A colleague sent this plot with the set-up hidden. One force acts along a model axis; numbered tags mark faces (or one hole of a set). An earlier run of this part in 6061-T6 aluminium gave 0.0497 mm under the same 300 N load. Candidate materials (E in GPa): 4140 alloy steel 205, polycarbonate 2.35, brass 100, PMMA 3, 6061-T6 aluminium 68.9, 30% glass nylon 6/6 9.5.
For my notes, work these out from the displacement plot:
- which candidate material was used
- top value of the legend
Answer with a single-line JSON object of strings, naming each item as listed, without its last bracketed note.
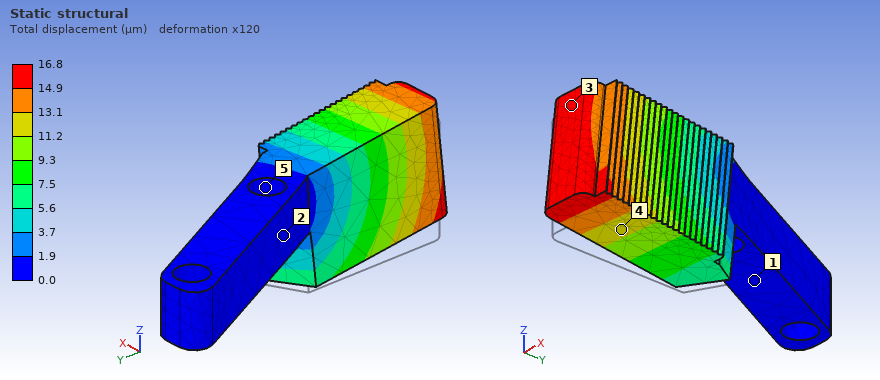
{"which candidate material was used": "4140 alloy steel", "top value of the legend": "16.8 µm"}
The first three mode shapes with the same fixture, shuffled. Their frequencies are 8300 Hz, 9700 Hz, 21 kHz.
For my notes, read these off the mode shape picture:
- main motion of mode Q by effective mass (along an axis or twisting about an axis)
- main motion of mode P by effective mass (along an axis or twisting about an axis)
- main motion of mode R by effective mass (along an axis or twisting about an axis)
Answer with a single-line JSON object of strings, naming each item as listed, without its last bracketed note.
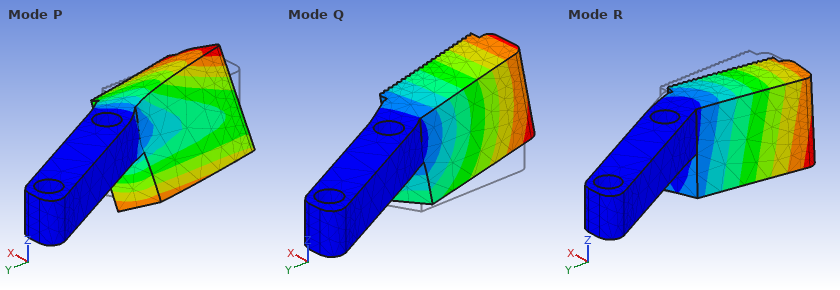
{"main motion of mode Q by effective mass": "along Z", "main motion of mode P by effective mass": "twisting about Y", "main motion of mode R by effective mass": "along X"}
